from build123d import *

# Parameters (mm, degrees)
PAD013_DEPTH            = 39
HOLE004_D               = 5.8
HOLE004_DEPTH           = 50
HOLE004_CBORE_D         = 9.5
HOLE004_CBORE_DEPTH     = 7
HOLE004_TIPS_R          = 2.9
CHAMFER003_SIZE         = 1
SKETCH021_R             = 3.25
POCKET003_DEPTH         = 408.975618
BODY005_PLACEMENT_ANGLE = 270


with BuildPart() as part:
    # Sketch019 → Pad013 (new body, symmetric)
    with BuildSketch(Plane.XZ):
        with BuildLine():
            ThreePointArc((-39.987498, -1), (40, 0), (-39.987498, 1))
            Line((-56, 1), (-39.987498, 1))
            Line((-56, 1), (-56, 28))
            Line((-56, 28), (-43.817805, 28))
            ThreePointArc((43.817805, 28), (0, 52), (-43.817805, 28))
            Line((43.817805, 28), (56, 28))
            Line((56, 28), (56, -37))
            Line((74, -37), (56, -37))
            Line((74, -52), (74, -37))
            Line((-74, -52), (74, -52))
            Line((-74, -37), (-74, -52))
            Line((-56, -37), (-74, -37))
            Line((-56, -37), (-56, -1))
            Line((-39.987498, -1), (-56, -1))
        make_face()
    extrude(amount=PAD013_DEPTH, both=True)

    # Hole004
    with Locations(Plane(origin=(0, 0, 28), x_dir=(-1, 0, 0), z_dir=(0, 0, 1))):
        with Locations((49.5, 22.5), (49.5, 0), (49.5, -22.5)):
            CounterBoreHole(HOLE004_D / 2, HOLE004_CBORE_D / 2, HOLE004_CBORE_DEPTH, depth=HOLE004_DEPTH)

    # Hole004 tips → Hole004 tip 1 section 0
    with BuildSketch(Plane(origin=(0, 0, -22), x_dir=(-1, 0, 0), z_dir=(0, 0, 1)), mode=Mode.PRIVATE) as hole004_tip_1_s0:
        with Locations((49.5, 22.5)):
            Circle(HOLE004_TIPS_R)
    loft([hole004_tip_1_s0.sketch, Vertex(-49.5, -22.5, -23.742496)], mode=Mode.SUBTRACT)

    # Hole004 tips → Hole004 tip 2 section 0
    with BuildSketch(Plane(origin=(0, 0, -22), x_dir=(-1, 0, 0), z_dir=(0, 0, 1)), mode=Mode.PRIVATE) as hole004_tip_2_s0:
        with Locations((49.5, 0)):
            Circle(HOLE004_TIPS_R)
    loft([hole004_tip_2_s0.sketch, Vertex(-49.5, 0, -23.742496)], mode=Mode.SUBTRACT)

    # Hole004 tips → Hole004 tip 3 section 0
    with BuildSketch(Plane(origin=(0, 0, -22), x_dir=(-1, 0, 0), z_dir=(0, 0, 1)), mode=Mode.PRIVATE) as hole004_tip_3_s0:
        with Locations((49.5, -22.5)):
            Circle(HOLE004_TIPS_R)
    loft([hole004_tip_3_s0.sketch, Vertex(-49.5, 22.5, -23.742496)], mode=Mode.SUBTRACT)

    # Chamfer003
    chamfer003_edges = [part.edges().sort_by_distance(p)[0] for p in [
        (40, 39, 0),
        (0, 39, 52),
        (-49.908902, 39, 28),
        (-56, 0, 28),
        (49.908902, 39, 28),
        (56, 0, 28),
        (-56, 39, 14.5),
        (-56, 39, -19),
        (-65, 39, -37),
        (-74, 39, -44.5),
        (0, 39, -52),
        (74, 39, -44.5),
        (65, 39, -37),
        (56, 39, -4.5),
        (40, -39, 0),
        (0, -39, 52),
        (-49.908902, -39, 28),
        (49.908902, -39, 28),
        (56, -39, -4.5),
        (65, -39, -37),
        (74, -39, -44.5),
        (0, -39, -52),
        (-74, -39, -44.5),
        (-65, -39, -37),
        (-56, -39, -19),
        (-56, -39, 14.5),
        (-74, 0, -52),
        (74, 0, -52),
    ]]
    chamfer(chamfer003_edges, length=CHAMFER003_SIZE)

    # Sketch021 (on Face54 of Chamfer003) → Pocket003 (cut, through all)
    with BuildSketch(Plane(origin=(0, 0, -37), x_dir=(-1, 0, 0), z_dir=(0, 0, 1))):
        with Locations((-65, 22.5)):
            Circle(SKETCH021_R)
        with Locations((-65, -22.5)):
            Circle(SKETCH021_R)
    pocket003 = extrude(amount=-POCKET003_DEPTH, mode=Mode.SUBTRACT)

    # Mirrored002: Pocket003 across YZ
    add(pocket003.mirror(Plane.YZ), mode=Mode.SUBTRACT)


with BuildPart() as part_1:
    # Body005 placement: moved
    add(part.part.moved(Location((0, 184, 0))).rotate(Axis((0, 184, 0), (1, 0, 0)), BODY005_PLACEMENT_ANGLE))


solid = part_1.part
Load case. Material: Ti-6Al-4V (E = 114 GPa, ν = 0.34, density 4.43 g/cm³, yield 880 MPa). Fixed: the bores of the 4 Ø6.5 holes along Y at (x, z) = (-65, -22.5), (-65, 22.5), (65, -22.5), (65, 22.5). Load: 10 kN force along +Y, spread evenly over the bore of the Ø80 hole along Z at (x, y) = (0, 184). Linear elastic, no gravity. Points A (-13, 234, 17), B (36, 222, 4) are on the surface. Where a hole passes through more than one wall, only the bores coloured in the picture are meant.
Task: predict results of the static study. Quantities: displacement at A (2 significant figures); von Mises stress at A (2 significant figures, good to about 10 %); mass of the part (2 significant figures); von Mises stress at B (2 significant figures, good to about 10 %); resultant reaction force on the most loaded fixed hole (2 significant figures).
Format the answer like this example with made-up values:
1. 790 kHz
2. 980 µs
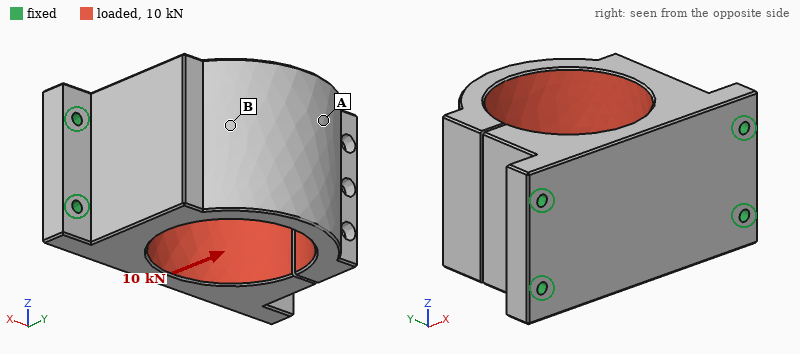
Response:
1. 0.59 mm
2. 17 MPa
3. 2.0 kg
4. 69 MPa
5. 2.7 kN
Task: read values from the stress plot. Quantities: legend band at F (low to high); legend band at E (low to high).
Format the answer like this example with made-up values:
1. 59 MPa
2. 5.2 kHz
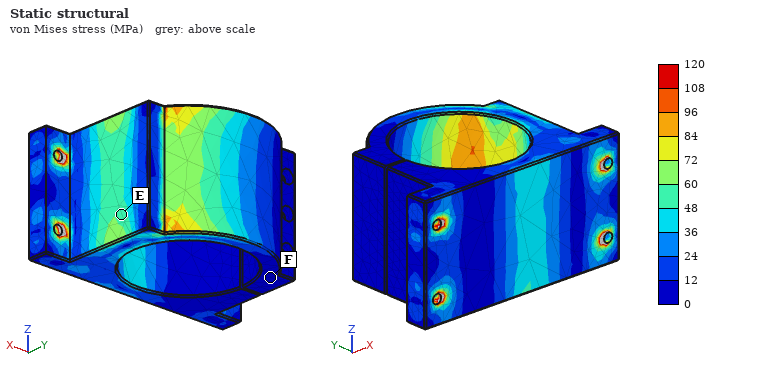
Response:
1. 0 to 12 MPa
2. 48 to 60 MPa
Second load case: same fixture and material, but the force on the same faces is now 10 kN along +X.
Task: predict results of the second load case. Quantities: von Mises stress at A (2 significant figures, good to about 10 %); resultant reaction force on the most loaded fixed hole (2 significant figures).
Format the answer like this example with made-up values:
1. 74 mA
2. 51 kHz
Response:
1. 18 MPa
2. 4.1 kN
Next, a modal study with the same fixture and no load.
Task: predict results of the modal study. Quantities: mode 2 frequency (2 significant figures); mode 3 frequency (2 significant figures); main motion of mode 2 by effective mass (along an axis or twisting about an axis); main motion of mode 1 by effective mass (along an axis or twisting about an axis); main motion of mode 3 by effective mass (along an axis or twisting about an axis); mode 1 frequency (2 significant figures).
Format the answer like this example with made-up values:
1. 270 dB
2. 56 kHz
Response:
1. 790 Hz
2. 1100 Hz
3. along Z
4. along Y
5. along X
6. 500 Hz
